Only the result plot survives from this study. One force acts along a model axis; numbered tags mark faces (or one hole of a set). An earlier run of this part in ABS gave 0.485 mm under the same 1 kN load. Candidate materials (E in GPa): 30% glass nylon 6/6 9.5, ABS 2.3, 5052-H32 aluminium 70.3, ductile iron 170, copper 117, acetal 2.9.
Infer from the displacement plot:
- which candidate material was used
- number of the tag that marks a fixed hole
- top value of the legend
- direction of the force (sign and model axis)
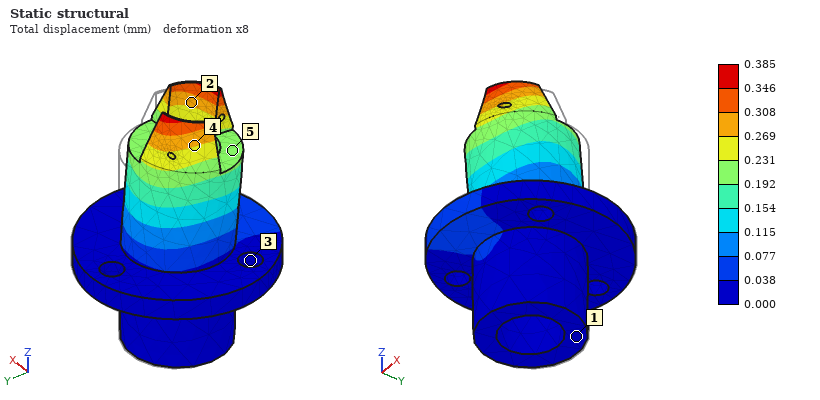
acetal
3
0.385 mm
-Y
